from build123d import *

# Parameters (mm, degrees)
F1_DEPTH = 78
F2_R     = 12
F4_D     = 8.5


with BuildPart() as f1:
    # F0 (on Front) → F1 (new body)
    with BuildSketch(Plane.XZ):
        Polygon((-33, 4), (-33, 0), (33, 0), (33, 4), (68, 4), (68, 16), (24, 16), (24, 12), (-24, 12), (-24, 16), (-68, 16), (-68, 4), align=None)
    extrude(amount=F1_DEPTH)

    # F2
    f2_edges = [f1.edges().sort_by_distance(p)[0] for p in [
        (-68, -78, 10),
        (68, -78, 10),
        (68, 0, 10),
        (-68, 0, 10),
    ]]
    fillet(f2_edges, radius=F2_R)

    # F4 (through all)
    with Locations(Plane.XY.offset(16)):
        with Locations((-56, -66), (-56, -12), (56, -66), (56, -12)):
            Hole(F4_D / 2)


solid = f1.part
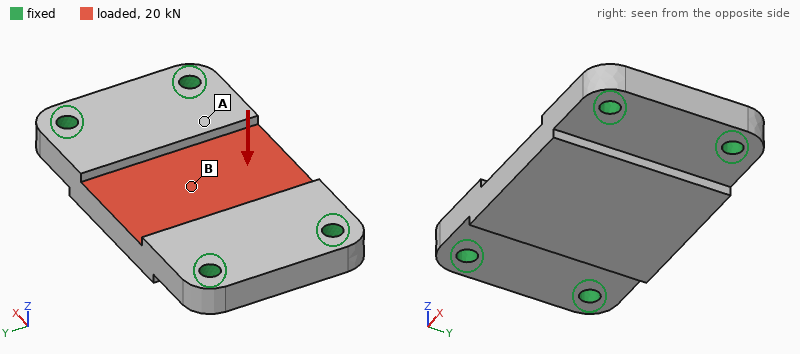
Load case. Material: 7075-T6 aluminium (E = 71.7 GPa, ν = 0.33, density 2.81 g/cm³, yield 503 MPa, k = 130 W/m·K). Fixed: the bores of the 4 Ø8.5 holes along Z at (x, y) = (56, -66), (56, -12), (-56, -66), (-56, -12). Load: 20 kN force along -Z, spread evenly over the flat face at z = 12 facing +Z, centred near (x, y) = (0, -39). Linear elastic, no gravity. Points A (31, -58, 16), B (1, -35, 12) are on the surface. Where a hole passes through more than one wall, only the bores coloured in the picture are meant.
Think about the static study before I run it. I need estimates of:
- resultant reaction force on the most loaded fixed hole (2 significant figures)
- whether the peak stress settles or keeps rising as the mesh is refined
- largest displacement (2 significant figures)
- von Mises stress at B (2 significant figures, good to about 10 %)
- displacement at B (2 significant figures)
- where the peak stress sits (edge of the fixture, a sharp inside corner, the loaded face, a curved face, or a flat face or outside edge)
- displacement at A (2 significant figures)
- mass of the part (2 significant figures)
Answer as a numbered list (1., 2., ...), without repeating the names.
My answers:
1. 8.8 kN
2. keeps rising
3. 0.16 mm
4. 56 MPa
5. 0.15 mm
6. edge of the fixture
7. 0.084 mm
8. 360 g
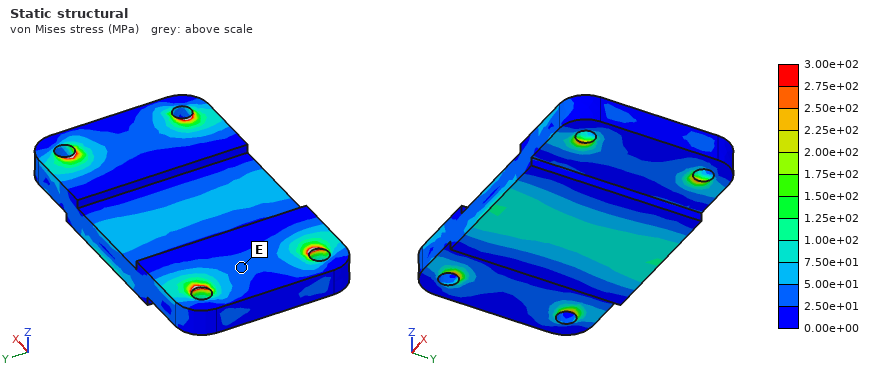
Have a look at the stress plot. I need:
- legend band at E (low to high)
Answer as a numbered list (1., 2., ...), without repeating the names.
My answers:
1. 2.50e+01 to 5.00e+01 MPa
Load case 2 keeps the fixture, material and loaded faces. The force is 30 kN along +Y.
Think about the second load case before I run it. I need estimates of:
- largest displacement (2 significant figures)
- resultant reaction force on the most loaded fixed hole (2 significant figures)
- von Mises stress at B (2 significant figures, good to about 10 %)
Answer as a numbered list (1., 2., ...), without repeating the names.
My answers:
1. 55 µm
2. 9.2 kN
3. 14 MPa
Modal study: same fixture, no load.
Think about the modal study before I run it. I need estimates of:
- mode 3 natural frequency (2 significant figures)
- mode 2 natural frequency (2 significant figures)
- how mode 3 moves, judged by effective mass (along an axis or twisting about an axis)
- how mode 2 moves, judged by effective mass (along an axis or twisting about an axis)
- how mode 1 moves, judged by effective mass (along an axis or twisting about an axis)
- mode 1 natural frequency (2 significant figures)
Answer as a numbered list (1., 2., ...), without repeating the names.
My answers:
1. 11 kHz
2. 6600 Hz
3. twisting about Y
4. twisting about X
5. along Z
6. 4700 Hz
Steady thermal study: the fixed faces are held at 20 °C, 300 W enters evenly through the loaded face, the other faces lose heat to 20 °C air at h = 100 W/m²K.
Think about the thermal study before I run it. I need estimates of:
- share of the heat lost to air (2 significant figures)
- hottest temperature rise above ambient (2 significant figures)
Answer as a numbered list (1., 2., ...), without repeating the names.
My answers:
1. 17 %
2. 53 K
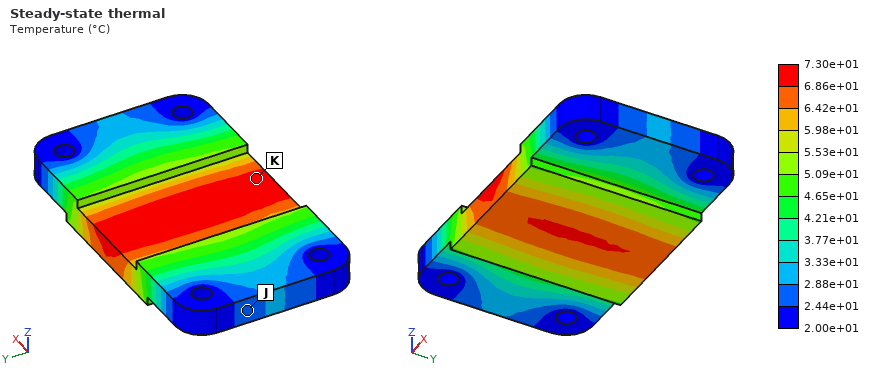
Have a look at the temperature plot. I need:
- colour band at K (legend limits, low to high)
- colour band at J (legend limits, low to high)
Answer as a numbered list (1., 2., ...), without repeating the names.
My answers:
1. 6.86e+01 to 7.30e+01 °C
2. 2.44e+01 to 2.88e+01 °C
